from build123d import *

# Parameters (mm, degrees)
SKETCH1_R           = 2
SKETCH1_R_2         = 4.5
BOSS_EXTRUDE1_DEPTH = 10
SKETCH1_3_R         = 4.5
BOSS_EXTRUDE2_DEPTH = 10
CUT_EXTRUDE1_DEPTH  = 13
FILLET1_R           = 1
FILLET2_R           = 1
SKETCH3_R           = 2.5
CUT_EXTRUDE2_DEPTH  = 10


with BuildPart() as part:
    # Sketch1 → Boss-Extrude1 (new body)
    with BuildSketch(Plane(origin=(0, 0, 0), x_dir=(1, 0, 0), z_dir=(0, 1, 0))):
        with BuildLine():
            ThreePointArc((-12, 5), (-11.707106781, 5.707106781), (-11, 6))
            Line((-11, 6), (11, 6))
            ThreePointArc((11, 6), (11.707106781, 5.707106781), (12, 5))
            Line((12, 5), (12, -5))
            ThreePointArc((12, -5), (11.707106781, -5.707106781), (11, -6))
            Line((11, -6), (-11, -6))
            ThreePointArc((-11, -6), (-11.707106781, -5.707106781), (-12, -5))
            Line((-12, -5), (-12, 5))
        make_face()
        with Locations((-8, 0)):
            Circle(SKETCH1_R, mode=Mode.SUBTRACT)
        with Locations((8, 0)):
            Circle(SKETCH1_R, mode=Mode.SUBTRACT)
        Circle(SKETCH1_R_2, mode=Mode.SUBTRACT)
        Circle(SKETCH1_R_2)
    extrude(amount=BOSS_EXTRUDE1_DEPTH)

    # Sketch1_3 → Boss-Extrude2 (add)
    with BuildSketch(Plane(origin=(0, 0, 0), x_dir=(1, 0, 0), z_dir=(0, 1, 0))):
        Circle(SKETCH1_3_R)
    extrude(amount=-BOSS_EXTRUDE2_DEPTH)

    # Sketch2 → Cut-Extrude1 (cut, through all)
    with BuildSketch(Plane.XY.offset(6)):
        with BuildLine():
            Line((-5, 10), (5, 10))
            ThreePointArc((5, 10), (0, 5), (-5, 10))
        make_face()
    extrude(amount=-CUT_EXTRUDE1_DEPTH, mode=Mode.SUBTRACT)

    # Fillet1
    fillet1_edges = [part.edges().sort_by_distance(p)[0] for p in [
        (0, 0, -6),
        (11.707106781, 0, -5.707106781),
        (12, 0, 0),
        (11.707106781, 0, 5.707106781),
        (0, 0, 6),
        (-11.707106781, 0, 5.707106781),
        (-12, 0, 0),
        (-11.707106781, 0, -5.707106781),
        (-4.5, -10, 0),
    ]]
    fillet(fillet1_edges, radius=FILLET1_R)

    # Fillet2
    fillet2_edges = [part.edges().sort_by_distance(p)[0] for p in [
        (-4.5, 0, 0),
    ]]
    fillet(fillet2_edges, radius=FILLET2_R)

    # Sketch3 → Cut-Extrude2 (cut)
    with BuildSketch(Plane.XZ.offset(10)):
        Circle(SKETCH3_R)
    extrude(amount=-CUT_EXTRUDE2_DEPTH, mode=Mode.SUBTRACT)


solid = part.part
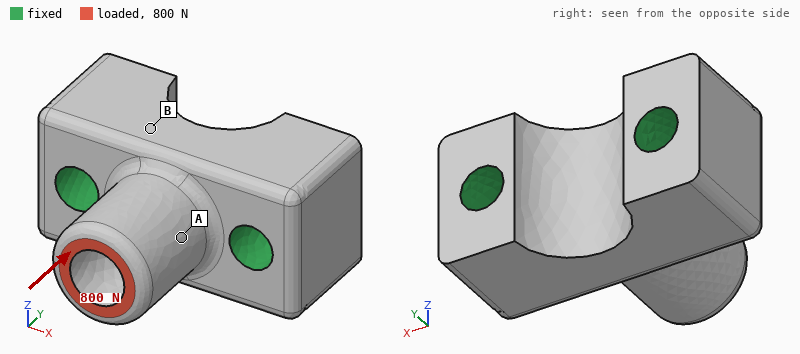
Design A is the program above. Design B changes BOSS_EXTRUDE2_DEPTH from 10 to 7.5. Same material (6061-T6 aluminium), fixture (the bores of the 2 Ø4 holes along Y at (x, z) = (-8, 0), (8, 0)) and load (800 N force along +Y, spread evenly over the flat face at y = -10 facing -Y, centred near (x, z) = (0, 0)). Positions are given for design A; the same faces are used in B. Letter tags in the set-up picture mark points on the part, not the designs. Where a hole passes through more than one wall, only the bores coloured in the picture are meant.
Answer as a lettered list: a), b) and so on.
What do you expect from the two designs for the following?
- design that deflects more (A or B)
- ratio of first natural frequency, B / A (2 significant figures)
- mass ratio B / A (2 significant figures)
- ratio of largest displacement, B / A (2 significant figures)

a) A
b) 1.4
c) 0.96
d) 0.86
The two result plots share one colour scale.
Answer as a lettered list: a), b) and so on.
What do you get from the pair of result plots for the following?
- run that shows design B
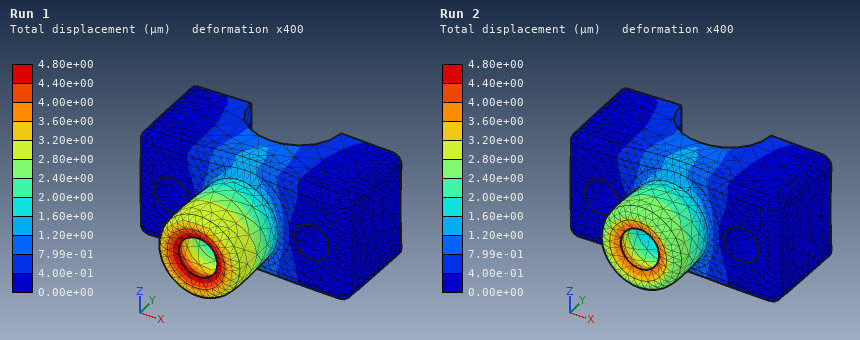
a) Run 2
